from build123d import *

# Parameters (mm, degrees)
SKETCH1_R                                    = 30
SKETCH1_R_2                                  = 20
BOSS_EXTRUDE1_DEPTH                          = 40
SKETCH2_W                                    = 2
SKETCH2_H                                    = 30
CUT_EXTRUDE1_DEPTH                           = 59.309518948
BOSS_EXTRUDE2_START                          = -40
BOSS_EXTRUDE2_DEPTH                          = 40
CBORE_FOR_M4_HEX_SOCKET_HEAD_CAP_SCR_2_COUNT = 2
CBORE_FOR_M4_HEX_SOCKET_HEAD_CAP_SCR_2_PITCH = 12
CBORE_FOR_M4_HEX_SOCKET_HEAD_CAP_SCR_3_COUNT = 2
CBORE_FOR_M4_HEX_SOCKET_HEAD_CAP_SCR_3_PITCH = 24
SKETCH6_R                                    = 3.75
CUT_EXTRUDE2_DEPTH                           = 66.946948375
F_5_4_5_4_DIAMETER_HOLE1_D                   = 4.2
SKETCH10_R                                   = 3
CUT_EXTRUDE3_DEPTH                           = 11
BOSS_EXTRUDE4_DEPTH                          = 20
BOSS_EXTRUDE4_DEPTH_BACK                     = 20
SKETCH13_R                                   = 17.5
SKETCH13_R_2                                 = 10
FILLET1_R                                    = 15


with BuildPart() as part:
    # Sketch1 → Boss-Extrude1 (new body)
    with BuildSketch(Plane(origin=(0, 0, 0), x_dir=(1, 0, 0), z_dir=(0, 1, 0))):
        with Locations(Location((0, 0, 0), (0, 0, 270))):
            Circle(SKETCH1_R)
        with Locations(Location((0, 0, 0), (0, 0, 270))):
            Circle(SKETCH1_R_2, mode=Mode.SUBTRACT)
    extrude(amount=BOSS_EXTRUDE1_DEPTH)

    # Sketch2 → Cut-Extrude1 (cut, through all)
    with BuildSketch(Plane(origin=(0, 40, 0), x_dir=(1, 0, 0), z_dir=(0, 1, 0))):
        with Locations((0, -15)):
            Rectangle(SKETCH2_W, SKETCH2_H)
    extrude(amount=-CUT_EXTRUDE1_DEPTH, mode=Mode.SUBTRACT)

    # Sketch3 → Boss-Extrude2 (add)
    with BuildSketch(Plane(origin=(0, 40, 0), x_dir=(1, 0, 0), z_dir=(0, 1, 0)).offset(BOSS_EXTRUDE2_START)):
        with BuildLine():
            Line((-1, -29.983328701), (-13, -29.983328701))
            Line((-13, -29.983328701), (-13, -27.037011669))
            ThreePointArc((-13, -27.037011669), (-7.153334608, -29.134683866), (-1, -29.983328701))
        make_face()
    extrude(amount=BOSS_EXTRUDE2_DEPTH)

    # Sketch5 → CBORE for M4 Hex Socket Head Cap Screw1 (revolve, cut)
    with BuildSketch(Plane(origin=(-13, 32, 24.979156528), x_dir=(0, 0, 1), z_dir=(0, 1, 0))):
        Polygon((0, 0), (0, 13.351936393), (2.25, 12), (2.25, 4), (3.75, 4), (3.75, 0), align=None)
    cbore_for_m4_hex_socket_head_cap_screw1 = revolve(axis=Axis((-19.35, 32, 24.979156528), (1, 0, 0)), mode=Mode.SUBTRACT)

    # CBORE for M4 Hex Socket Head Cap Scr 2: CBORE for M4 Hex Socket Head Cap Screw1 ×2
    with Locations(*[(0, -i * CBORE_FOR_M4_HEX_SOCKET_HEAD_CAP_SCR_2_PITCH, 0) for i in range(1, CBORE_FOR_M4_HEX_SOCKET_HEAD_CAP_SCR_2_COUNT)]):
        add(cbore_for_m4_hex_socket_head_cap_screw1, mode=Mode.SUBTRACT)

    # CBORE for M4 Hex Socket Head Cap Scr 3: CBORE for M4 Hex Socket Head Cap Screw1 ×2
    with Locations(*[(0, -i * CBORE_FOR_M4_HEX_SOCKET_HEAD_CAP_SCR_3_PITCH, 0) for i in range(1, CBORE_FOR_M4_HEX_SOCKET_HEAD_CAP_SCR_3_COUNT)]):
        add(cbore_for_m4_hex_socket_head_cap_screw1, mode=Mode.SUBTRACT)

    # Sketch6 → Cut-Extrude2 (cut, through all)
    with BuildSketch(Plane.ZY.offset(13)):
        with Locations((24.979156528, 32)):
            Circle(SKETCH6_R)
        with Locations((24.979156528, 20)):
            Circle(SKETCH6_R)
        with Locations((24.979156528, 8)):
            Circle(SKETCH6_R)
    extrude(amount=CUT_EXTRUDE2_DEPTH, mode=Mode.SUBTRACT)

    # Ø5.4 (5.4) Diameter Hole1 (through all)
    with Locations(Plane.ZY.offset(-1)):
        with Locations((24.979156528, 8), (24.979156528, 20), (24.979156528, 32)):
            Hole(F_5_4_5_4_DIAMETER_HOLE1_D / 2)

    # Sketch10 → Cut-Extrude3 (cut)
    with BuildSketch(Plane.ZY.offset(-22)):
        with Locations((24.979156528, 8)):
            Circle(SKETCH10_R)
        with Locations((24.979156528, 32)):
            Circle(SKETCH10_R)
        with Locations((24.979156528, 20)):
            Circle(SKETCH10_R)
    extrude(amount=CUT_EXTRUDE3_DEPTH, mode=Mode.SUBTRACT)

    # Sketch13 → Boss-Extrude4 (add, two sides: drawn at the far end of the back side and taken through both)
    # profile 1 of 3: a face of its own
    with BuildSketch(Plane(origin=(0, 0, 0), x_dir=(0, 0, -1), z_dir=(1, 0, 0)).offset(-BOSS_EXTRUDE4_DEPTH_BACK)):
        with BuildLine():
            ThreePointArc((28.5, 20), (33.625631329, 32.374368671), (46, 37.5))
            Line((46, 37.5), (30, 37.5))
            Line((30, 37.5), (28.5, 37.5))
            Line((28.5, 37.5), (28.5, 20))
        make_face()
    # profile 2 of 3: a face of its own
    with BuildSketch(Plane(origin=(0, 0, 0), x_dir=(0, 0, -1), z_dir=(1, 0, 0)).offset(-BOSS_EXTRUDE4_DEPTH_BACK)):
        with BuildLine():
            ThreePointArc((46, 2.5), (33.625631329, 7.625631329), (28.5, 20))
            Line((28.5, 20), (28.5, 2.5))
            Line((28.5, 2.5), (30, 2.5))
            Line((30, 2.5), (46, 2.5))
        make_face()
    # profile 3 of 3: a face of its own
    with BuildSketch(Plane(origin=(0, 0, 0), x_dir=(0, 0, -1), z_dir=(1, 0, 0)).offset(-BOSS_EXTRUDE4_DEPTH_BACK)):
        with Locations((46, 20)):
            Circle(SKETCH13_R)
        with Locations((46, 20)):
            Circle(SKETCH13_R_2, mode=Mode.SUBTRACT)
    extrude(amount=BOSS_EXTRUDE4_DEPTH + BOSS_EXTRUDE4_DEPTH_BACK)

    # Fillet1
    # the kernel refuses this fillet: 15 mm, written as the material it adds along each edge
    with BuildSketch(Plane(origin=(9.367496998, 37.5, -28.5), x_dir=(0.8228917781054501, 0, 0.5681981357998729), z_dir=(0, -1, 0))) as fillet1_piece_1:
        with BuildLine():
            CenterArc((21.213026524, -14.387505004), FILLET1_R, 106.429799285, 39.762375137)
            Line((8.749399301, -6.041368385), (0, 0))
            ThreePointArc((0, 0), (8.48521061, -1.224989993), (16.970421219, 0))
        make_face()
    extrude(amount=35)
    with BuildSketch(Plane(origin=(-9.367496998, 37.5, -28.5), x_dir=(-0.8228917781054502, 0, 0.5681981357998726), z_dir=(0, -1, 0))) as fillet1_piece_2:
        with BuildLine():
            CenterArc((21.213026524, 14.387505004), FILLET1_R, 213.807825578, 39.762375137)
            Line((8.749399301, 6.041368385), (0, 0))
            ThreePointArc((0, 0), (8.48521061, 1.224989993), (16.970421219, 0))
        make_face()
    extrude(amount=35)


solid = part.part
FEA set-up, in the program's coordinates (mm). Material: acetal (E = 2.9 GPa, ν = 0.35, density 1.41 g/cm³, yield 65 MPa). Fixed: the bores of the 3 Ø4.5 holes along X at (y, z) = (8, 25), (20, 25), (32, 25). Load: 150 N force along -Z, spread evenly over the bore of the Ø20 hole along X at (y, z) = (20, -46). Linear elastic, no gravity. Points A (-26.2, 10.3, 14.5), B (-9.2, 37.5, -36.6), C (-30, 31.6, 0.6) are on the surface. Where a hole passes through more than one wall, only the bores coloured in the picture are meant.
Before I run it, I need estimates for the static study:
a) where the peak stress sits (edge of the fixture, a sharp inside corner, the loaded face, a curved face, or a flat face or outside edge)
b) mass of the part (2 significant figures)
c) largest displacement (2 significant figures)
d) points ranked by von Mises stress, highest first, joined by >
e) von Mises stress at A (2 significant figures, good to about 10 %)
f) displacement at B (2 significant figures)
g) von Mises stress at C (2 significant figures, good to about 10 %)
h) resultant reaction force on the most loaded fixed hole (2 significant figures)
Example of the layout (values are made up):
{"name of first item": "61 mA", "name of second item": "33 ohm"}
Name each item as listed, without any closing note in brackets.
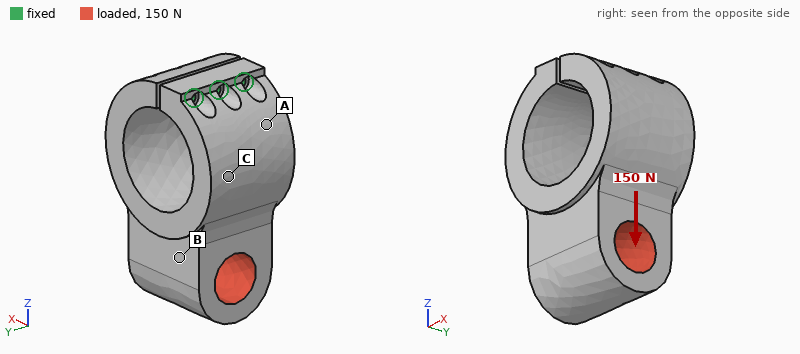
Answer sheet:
{"where the peak stress sits": "a curved face", "mass of the part": "130 g", "largest displacement": "1.4 mm", "points ranked by von Mises stress, highest first, joined by >": "C > A > B", "von Mises stress at A": "3.5 MPa", "displacement at B": "0.73 mm", "von Mises stress at C": "4.3 MPa", "resultant reaction force on the most loaded fixed hole": "61 N"}
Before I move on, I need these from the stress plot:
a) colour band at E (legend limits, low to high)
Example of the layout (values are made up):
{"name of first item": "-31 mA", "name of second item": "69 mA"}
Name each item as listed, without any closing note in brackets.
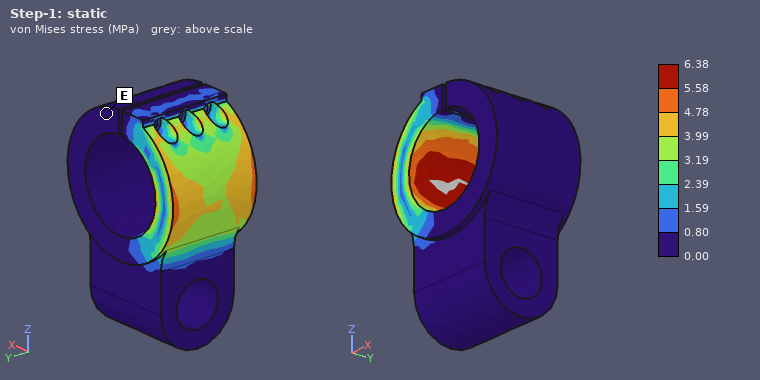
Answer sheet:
{"colour band at E": "0.00 to 0.80 MPa"}
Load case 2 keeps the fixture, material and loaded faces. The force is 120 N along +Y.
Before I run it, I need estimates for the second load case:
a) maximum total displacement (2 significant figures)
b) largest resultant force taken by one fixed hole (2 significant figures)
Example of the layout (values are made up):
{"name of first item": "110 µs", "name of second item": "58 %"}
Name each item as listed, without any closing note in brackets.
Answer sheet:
{"maximum total displacement": "1.3 mm", "largest resultant force taken by one fixed hole": "290 N"}
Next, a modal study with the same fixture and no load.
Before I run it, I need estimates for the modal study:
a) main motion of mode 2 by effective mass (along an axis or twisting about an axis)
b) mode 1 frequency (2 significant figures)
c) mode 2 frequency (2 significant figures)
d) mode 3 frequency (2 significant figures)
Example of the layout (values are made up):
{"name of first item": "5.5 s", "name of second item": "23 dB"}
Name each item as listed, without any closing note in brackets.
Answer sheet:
{"main motion of mode 2 by effective mass": "along Y", "mode 1 frequency": "130 Hz", "mode 2 frequency": "200 Hz", "mode 3 frequency": "380 Hz"}
